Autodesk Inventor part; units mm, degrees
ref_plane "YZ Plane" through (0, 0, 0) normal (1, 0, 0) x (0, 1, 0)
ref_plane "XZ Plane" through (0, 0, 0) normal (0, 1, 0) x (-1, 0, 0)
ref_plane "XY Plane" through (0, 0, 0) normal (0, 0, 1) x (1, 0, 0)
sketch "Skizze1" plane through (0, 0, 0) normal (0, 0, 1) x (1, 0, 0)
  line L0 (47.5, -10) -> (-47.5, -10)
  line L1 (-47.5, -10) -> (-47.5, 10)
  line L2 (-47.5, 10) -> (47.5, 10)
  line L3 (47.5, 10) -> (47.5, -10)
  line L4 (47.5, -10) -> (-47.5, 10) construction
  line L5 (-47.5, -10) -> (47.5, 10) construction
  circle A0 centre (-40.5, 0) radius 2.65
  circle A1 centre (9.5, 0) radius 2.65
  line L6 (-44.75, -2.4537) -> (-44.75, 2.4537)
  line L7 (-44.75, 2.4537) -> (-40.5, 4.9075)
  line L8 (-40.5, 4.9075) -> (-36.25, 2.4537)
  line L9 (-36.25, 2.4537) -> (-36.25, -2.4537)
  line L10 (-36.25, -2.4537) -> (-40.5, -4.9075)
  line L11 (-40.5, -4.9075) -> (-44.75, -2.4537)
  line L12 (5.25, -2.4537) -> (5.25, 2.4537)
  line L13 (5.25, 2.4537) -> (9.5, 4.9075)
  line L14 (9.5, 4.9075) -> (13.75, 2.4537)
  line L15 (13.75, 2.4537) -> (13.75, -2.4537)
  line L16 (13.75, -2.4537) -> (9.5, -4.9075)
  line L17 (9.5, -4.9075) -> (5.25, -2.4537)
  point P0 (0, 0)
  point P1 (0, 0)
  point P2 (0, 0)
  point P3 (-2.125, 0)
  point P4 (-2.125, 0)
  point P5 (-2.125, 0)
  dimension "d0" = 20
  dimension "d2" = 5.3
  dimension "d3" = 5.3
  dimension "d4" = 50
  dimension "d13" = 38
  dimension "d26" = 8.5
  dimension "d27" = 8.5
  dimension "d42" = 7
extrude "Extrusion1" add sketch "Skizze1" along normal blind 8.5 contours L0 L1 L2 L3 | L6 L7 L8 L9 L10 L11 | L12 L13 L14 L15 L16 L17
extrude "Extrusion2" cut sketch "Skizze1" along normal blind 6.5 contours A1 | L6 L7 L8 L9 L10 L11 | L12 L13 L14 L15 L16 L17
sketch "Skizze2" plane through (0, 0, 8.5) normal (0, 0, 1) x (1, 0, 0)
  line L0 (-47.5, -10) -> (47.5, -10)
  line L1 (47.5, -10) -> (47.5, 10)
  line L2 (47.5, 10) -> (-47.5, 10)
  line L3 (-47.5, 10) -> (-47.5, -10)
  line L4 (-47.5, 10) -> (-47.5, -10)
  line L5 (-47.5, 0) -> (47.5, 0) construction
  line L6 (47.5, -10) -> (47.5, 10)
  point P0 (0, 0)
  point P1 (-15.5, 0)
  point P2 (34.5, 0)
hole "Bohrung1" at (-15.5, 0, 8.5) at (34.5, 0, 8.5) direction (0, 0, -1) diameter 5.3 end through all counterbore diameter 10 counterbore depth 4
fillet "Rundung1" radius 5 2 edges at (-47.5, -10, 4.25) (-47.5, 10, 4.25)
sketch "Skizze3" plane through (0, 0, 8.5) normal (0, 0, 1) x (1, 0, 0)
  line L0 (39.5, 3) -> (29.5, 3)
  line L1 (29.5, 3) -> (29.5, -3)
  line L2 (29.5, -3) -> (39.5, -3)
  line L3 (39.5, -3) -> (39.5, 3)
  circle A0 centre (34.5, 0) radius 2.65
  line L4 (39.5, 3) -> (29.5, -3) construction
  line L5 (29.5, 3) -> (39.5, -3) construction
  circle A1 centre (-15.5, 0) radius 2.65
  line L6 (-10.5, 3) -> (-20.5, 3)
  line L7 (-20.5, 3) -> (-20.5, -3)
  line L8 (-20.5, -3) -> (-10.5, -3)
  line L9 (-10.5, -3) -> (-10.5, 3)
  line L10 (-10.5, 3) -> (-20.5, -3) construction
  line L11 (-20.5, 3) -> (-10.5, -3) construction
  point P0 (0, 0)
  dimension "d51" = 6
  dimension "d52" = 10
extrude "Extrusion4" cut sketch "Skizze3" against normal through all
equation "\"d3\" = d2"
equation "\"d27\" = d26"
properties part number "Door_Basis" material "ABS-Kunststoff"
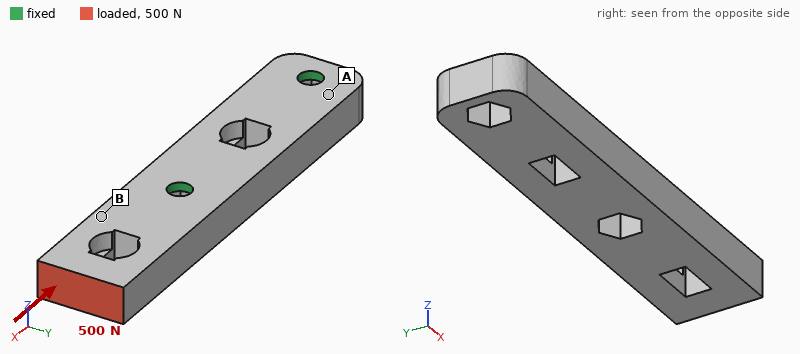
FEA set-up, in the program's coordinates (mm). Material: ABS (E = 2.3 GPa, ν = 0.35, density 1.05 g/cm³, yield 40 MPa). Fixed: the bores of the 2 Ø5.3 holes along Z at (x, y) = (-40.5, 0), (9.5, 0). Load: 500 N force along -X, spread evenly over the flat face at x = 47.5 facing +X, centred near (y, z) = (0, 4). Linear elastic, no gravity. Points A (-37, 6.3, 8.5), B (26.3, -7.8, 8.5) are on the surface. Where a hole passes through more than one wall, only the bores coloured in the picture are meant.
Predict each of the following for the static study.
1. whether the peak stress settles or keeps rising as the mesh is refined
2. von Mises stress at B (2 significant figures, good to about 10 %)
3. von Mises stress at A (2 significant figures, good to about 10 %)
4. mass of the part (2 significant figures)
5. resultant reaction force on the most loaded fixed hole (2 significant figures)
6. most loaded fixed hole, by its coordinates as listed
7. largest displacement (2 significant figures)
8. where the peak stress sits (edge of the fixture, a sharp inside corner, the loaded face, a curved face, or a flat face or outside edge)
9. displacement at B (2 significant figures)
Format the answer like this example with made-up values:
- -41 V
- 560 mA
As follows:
- keeps rising
- 4.4 MPa
- 1.5 MPa
- 15 g
- 350 N
- (9.5, 0)
- 0.29 mm
- edge of the fixture
- 0.12 mm
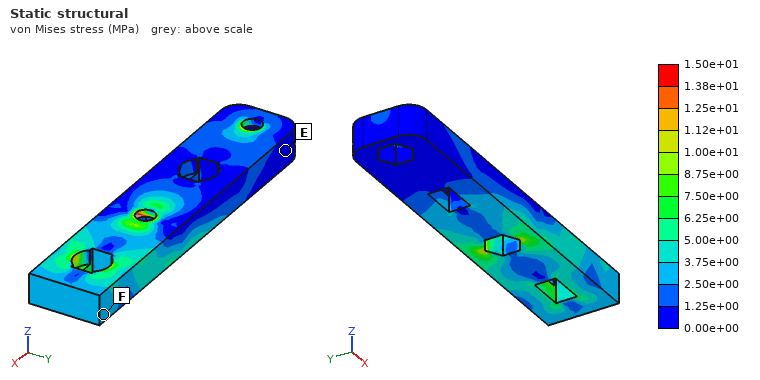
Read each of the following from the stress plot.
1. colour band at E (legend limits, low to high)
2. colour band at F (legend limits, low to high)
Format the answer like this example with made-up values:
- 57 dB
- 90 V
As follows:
- 0.00e+00 to 1.25e+00 MPa
- 2.50e+00 to 3.75e+00 MPa
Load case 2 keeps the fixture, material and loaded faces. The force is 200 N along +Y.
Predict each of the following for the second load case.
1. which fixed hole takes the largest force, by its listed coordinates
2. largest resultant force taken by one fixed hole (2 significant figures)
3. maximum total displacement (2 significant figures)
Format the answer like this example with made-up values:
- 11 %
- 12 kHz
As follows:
- (9.5, 0)
- 320 N
- 0.94 mm
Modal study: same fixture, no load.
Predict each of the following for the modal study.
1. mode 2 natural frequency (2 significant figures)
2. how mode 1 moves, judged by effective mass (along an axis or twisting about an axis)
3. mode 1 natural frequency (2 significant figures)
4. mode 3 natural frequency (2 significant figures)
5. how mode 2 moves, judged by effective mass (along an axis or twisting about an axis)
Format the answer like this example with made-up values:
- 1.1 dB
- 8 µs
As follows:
- 1600 Hz
- along Z
- 1000 Hz
- 2100 Hz
- along Y
